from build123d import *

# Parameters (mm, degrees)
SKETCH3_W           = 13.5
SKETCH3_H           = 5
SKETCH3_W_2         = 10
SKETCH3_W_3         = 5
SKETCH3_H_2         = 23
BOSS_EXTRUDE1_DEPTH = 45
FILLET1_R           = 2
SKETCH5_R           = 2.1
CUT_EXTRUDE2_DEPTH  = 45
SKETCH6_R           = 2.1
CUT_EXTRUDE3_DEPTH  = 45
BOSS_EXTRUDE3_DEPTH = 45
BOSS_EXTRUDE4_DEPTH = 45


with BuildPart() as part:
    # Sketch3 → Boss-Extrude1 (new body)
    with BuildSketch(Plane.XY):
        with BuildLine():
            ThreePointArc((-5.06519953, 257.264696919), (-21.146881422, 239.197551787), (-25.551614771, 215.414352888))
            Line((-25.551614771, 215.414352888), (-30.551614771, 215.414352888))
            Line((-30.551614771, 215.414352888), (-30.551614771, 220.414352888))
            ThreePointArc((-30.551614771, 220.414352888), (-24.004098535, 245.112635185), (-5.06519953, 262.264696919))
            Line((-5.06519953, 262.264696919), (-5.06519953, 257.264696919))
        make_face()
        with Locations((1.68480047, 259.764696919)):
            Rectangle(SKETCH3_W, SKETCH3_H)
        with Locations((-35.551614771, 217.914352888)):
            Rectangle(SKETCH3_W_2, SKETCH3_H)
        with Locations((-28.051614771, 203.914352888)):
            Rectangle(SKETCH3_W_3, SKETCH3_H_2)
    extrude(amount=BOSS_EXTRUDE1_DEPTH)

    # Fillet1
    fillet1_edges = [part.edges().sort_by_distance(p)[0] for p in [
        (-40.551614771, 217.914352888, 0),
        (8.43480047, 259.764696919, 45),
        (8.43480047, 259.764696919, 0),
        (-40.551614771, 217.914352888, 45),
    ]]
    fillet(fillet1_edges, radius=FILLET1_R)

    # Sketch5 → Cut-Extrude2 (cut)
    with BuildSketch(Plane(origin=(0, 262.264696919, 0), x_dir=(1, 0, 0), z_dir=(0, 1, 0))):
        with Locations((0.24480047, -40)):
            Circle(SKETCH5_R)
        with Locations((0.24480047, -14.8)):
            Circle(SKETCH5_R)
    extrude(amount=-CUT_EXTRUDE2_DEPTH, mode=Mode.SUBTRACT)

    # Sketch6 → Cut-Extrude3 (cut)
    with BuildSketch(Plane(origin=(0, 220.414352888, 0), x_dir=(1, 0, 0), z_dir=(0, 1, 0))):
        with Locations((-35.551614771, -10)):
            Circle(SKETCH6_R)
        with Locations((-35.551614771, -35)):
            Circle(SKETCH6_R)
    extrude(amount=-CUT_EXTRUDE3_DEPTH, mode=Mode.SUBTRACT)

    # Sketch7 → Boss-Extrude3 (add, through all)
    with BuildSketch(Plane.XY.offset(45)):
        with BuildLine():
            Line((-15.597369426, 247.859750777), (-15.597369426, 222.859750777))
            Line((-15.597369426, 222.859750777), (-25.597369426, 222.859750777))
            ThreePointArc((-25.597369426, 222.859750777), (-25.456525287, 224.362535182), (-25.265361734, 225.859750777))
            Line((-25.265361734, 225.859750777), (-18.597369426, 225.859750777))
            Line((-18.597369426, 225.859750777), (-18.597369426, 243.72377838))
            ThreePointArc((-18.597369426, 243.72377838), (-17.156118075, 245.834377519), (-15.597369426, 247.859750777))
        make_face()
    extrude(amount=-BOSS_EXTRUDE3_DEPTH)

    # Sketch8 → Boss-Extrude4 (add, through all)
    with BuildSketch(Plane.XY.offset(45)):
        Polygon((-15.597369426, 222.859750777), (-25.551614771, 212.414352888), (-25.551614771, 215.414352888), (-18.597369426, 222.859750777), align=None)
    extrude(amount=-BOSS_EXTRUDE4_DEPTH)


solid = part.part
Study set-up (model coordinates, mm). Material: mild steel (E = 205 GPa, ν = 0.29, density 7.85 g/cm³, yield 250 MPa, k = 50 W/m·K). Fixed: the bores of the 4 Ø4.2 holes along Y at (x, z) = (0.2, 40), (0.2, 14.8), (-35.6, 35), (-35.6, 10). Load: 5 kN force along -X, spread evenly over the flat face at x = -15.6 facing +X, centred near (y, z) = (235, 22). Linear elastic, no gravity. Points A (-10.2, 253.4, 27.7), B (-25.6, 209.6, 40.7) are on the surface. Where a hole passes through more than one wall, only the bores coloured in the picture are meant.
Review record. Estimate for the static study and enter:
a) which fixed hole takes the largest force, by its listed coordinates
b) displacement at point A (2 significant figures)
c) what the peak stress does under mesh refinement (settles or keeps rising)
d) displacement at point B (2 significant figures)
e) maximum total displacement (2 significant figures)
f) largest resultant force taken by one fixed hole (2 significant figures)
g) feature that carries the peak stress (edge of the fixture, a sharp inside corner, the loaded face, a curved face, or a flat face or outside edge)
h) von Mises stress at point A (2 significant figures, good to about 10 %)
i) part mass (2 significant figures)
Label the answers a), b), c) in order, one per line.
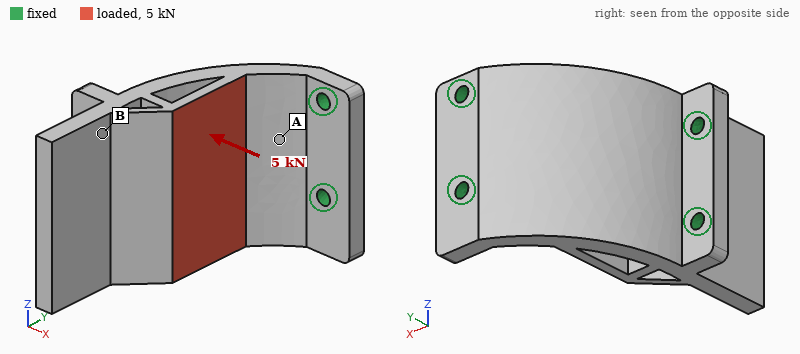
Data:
a) (0.2, 14.8)
b) 4.6 µm
c) keeps rising
d) 4.5 µm
e) 18 µm
f) 2.1 kN
g) edge of the fixture
h) 26 MPa
i) 220 g
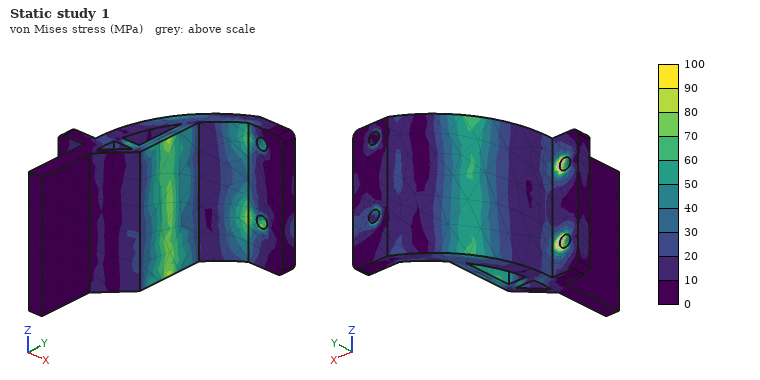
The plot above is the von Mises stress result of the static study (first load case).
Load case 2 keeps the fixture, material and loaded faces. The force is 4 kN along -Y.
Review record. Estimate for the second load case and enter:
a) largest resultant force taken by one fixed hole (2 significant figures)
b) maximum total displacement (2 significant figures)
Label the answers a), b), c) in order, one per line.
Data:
a) 2.0 kN
b) 17 µm
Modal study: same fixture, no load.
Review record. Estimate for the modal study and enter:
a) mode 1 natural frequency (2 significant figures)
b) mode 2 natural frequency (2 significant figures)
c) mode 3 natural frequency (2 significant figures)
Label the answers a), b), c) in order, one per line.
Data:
a) 6200 Hz
b) 9600 Hz
c) 11 kHz
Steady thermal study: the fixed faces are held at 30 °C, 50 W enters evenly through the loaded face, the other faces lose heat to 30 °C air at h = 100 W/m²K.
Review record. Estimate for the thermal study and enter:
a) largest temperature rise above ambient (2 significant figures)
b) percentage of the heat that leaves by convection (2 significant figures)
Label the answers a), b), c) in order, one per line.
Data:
a) 47 K
b) 43 %
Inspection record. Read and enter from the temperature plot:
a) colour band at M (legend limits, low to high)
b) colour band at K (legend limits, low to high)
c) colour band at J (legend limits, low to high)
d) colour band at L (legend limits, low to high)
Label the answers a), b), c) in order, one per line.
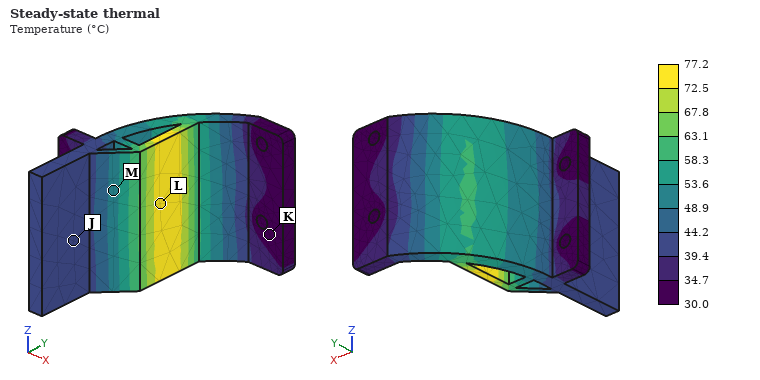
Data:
a) 48.9 to 53.6 °C
b) 30.0 to 34.7 °C
c) 39.4 to 44.2 °C
d) 72.5 to 77.2 °C
